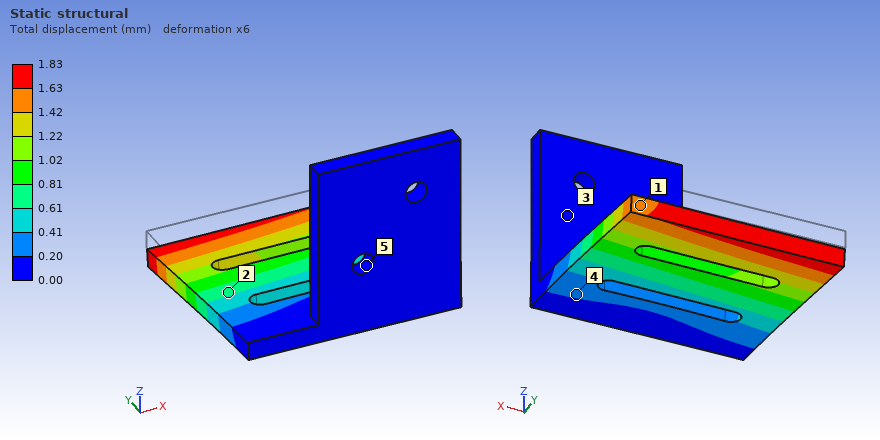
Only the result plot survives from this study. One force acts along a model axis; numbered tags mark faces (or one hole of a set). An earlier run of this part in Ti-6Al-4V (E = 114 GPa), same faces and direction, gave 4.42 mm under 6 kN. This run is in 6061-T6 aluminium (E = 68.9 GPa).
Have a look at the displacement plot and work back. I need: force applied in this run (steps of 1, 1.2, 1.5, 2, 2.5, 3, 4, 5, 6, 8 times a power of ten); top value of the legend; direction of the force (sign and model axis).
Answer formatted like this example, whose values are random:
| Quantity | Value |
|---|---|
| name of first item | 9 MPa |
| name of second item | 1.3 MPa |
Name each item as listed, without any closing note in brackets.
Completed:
| Quantity | Value |
|---|---|
| force applied in this run | 1.5 kN |
| top value of the legend | 1.83 mm |
| direction of the force | -Z |
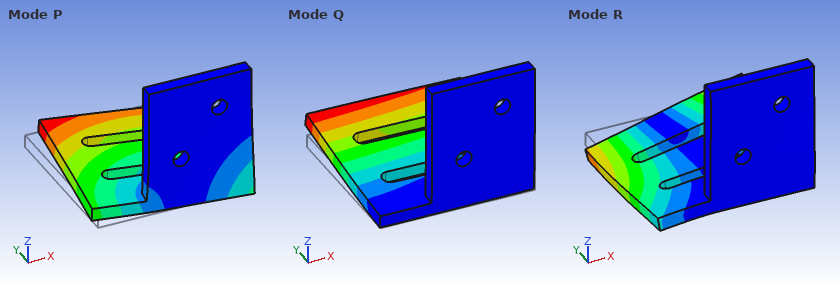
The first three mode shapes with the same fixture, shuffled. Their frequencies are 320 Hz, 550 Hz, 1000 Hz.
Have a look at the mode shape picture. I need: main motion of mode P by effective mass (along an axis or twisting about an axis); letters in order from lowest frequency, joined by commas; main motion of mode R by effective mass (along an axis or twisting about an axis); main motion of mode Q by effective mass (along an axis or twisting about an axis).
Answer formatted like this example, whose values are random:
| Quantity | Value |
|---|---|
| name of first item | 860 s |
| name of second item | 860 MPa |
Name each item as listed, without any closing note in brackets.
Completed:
| Quantity | Value |
|---|---|
| main motion of mode P by effective mass | along X |
| letters in order from lowest frequency, joined by commas | Q, P, R |
| main motion of mode R by effective mass | twisting about Y |
| main motion of mode Q by effective mass | along Z |
